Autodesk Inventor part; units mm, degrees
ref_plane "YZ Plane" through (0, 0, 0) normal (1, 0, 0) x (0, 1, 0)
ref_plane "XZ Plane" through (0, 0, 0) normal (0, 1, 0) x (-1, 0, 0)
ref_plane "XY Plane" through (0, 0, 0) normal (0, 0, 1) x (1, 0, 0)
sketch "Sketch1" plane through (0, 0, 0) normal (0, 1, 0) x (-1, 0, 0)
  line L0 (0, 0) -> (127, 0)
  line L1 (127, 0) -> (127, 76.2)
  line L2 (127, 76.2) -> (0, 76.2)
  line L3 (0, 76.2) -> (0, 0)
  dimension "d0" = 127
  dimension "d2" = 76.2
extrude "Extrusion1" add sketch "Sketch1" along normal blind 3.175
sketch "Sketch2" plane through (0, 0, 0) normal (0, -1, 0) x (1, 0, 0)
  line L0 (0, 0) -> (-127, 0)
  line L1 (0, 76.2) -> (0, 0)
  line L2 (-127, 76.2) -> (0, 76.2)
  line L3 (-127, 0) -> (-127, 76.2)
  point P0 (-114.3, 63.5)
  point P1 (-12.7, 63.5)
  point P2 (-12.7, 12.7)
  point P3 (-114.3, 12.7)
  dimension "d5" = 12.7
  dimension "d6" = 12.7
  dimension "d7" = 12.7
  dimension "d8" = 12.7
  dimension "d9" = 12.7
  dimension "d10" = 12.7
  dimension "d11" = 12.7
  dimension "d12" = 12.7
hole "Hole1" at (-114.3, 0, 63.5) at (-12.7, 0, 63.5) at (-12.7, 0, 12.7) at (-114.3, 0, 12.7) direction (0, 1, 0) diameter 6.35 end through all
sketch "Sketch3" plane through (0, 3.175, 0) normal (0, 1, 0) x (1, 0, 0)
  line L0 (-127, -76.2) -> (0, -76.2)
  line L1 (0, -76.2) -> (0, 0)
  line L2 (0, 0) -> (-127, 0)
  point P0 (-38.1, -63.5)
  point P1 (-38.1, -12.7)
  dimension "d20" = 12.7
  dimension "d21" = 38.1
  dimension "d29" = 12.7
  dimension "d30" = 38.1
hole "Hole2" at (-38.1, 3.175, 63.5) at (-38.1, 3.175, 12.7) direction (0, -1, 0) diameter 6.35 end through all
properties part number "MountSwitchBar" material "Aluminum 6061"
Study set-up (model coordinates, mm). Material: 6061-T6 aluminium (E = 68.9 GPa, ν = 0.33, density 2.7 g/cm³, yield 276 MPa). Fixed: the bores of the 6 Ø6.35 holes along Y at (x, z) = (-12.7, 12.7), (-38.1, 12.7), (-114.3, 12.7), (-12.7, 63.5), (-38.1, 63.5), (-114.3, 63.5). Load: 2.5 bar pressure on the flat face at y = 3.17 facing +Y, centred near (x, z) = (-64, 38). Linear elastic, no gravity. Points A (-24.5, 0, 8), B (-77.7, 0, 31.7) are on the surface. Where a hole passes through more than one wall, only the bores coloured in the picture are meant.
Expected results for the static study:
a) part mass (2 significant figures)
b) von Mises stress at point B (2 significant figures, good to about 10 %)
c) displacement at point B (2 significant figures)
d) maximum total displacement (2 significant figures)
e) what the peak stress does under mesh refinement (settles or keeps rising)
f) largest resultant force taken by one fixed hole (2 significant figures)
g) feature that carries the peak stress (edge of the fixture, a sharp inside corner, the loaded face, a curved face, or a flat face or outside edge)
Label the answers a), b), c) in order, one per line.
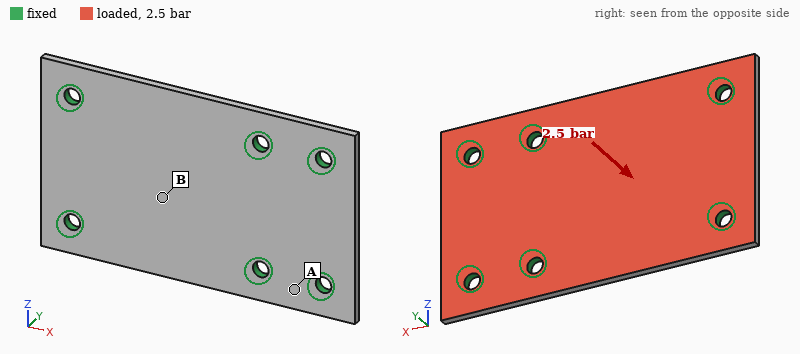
a) 81 g
b) 31 MPa
c) 0.13 mm
d) 0.13 mm
e) keeps rising
f) 510 N
g) edge of the fixture
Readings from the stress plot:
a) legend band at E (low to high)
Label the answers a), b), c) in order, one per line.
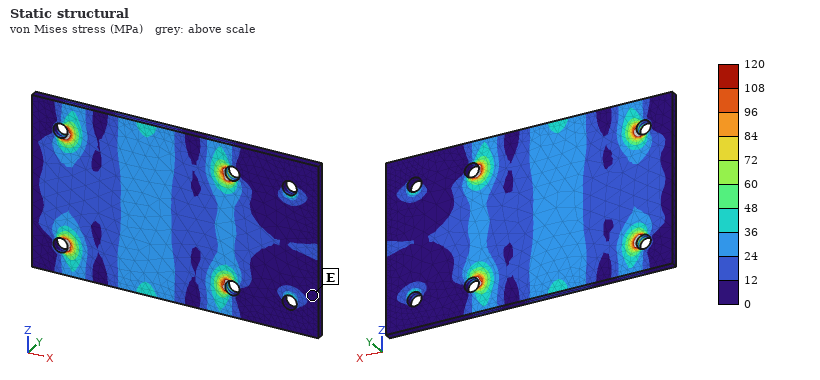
a) 0 to 12 MPa
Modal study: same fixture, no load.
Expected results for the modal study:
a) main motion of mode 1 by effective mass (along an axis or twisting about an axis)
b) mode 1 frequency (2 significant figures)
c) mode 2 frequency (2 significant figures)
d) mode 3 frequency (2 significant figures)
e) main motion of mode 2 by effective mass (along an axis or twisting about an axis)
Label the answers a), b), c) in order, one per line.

a) along Y
b) 2800 Hz
c) 3500 Hz
d) 4900 Hz
e) twisting about X
